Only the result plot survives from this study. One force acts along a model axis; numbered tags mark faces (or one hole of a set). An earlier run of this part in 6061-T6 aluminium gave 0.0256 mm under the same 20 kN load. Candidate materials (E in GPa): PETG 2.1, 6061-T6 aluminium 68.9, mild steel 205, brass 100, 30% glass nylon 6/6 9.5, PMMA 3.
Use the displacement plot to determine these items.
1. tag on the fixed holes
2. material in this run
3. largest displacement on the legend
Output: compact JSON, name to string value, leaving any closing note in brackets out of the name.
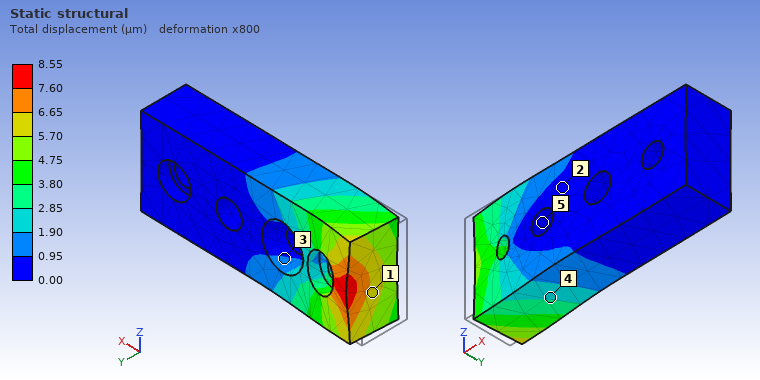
{"tag on the fixed holes": "5", "material in this run": "mild steel", "largest displacement on the legend": "8.55 µm"}
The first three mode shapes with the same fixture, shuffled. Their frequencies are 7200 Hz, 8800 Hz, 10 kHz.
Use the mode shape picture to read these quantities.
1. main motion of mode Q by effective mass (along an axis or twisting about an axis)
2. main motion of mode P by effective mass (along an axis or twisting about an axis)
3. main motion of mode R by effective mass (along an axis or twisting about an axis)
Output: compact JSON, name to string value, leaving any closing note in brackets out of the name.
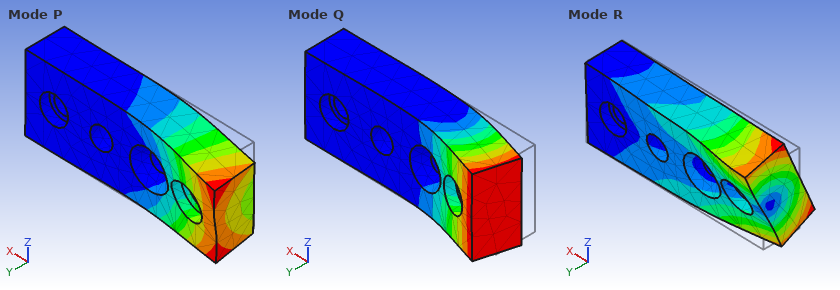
{"main motion of mode Q by effective mass": "along Y", "main motion of mode P by effective mass": "along Z", "main motion of mode R by effective mass": "twisting about X"}
